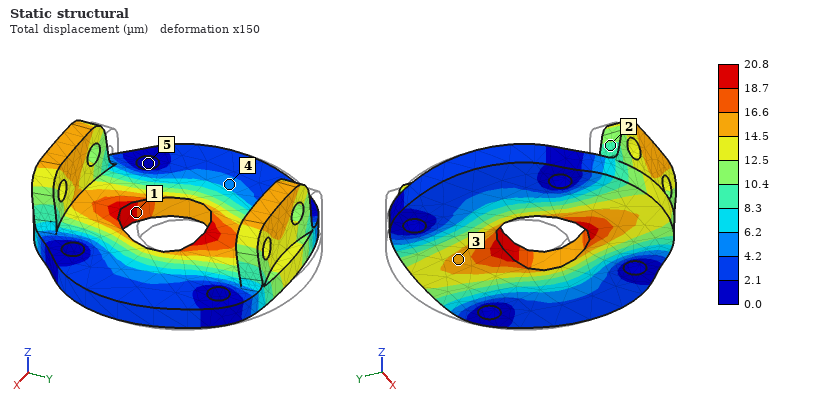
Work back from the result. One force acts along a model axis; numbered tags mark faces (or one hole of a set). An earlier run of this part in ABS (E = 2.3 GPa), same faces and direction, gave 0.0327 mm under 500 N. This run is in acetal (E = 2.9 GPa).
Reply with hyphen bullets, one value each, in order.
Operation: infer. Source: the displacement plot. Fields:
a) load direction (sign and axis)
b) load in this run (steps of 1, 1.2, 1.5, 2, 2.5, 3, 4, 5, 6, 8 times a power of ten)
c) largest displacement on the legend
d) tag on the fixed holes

- -Y
- 400 N
- 20.8 µm
- 5
